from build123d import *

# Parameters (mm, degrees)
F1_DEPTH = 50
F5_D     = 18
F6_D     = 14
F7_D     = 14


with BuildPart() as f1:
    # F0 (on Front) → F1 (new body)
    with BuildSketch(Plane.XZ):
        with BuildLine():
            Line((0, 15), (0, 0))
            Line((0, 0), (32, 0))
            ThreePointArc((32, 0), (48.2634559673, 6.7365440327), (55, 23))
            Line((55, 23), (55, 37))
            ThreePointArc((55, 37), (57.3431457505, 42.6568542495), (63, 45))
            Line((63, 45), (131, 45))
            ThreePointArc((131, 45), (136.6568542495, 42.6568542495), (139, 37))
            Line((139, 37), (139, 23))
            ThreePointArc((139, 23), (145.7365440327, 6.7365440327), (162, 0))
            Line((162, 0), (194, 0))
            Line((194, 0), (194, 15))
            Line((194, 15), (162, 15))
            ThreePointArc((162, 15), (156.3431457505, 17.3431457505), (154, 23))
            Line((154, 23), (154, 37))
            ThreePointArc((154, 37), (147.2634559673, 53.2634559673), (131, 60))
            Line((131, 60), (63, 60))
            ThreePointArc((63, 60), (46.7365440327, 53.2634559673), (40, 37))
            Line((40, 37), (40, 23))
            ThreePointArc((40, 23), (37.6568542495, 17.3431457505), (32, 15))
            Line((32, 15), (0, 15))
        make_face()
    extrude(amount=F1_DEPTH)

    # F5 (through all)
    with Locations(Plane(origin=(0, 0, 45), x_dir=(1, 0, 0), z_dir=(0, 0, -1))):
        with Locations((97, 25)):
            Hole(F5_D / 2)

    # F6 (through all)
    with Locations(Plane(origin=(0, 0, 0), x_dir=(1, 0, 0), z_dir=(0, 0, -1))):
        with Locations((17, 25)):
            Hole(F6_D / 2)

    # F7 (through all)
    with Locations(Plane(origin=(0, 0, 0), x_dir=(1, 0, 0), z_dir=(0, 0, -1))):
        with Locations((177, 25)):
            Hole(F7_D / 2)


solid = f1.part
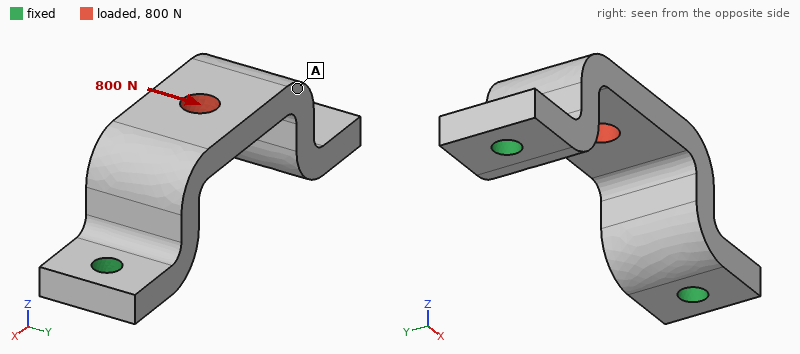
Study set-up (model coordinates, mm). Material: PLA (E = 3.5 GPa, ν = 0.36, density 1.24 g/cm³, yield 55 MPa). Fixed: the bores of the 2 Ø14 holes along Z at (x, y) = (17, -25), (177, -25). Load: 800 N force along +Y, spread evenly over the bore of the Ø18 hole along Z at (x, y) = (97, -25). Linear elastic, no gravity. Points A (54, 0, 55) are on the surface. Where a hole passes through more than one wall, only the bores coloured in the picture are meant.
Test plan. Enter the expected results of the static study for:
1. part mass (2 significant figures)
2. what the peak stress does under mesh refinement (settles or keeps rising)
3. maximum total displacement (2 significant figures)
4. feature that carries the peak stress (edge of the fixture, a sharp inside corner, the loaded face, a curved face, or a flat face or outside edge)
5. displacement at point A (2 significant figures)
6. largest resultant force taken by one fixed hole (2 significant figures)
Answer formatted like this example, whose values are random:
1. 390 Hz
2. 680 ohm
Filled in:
1. 230 g
2. keeps rising
3. 0.44 mm
4. edge of the fixture
5. 0.37 mm
6. 400 N
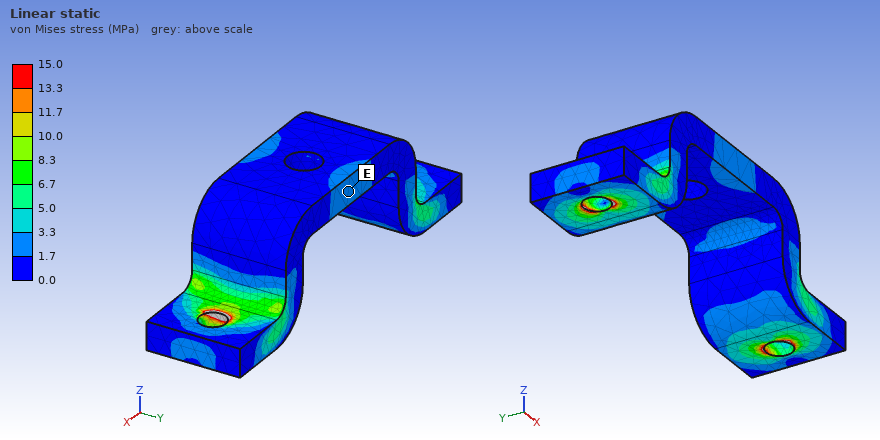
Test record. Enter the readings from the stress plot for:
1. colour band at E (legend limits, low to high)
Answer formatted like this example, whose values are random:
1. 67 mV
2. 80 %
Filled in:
1. 1.7 to 3.3 MPa
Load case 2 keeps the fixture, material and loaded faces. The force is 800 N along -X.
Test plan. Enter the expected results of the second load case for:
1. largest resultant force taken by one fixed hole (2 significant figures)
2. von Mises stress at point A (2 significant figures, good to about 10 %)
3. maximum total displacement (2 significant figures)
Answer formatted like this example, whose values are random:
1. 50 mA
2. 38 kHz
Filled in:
1. 450 N
2. 2.1 MPa
3. 0.15 mm
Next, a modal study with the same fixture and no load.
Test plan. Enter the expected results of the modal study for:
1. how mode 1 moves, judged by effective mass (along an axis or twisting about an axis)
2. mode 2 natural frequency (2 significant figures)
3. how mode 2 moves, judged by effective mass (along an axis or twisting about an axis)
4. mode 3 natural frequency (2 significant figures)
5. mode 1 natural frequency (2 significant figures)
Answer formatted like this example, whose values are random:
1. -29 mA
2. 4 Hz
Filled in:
1. along Y
2. 1100 Hz
3. along X
4. 1400 Hz
5. 720 Hz
